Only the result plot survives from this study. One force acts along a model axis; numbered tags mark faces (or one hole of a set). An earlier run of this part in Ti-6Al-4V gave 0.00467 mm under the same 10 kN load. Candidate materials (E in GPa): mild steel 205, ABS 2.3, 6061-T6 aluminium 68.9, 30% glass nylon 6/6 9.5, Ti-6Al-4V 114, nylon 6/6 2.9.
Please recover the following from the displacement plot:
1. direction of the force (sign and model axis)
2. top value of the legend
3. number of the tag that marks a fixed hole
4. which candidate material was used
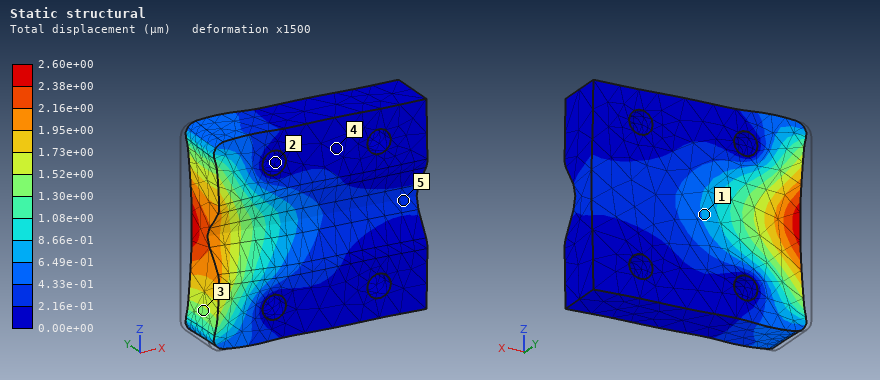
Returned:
+X
2.60e+00 µm
2
mild steel
